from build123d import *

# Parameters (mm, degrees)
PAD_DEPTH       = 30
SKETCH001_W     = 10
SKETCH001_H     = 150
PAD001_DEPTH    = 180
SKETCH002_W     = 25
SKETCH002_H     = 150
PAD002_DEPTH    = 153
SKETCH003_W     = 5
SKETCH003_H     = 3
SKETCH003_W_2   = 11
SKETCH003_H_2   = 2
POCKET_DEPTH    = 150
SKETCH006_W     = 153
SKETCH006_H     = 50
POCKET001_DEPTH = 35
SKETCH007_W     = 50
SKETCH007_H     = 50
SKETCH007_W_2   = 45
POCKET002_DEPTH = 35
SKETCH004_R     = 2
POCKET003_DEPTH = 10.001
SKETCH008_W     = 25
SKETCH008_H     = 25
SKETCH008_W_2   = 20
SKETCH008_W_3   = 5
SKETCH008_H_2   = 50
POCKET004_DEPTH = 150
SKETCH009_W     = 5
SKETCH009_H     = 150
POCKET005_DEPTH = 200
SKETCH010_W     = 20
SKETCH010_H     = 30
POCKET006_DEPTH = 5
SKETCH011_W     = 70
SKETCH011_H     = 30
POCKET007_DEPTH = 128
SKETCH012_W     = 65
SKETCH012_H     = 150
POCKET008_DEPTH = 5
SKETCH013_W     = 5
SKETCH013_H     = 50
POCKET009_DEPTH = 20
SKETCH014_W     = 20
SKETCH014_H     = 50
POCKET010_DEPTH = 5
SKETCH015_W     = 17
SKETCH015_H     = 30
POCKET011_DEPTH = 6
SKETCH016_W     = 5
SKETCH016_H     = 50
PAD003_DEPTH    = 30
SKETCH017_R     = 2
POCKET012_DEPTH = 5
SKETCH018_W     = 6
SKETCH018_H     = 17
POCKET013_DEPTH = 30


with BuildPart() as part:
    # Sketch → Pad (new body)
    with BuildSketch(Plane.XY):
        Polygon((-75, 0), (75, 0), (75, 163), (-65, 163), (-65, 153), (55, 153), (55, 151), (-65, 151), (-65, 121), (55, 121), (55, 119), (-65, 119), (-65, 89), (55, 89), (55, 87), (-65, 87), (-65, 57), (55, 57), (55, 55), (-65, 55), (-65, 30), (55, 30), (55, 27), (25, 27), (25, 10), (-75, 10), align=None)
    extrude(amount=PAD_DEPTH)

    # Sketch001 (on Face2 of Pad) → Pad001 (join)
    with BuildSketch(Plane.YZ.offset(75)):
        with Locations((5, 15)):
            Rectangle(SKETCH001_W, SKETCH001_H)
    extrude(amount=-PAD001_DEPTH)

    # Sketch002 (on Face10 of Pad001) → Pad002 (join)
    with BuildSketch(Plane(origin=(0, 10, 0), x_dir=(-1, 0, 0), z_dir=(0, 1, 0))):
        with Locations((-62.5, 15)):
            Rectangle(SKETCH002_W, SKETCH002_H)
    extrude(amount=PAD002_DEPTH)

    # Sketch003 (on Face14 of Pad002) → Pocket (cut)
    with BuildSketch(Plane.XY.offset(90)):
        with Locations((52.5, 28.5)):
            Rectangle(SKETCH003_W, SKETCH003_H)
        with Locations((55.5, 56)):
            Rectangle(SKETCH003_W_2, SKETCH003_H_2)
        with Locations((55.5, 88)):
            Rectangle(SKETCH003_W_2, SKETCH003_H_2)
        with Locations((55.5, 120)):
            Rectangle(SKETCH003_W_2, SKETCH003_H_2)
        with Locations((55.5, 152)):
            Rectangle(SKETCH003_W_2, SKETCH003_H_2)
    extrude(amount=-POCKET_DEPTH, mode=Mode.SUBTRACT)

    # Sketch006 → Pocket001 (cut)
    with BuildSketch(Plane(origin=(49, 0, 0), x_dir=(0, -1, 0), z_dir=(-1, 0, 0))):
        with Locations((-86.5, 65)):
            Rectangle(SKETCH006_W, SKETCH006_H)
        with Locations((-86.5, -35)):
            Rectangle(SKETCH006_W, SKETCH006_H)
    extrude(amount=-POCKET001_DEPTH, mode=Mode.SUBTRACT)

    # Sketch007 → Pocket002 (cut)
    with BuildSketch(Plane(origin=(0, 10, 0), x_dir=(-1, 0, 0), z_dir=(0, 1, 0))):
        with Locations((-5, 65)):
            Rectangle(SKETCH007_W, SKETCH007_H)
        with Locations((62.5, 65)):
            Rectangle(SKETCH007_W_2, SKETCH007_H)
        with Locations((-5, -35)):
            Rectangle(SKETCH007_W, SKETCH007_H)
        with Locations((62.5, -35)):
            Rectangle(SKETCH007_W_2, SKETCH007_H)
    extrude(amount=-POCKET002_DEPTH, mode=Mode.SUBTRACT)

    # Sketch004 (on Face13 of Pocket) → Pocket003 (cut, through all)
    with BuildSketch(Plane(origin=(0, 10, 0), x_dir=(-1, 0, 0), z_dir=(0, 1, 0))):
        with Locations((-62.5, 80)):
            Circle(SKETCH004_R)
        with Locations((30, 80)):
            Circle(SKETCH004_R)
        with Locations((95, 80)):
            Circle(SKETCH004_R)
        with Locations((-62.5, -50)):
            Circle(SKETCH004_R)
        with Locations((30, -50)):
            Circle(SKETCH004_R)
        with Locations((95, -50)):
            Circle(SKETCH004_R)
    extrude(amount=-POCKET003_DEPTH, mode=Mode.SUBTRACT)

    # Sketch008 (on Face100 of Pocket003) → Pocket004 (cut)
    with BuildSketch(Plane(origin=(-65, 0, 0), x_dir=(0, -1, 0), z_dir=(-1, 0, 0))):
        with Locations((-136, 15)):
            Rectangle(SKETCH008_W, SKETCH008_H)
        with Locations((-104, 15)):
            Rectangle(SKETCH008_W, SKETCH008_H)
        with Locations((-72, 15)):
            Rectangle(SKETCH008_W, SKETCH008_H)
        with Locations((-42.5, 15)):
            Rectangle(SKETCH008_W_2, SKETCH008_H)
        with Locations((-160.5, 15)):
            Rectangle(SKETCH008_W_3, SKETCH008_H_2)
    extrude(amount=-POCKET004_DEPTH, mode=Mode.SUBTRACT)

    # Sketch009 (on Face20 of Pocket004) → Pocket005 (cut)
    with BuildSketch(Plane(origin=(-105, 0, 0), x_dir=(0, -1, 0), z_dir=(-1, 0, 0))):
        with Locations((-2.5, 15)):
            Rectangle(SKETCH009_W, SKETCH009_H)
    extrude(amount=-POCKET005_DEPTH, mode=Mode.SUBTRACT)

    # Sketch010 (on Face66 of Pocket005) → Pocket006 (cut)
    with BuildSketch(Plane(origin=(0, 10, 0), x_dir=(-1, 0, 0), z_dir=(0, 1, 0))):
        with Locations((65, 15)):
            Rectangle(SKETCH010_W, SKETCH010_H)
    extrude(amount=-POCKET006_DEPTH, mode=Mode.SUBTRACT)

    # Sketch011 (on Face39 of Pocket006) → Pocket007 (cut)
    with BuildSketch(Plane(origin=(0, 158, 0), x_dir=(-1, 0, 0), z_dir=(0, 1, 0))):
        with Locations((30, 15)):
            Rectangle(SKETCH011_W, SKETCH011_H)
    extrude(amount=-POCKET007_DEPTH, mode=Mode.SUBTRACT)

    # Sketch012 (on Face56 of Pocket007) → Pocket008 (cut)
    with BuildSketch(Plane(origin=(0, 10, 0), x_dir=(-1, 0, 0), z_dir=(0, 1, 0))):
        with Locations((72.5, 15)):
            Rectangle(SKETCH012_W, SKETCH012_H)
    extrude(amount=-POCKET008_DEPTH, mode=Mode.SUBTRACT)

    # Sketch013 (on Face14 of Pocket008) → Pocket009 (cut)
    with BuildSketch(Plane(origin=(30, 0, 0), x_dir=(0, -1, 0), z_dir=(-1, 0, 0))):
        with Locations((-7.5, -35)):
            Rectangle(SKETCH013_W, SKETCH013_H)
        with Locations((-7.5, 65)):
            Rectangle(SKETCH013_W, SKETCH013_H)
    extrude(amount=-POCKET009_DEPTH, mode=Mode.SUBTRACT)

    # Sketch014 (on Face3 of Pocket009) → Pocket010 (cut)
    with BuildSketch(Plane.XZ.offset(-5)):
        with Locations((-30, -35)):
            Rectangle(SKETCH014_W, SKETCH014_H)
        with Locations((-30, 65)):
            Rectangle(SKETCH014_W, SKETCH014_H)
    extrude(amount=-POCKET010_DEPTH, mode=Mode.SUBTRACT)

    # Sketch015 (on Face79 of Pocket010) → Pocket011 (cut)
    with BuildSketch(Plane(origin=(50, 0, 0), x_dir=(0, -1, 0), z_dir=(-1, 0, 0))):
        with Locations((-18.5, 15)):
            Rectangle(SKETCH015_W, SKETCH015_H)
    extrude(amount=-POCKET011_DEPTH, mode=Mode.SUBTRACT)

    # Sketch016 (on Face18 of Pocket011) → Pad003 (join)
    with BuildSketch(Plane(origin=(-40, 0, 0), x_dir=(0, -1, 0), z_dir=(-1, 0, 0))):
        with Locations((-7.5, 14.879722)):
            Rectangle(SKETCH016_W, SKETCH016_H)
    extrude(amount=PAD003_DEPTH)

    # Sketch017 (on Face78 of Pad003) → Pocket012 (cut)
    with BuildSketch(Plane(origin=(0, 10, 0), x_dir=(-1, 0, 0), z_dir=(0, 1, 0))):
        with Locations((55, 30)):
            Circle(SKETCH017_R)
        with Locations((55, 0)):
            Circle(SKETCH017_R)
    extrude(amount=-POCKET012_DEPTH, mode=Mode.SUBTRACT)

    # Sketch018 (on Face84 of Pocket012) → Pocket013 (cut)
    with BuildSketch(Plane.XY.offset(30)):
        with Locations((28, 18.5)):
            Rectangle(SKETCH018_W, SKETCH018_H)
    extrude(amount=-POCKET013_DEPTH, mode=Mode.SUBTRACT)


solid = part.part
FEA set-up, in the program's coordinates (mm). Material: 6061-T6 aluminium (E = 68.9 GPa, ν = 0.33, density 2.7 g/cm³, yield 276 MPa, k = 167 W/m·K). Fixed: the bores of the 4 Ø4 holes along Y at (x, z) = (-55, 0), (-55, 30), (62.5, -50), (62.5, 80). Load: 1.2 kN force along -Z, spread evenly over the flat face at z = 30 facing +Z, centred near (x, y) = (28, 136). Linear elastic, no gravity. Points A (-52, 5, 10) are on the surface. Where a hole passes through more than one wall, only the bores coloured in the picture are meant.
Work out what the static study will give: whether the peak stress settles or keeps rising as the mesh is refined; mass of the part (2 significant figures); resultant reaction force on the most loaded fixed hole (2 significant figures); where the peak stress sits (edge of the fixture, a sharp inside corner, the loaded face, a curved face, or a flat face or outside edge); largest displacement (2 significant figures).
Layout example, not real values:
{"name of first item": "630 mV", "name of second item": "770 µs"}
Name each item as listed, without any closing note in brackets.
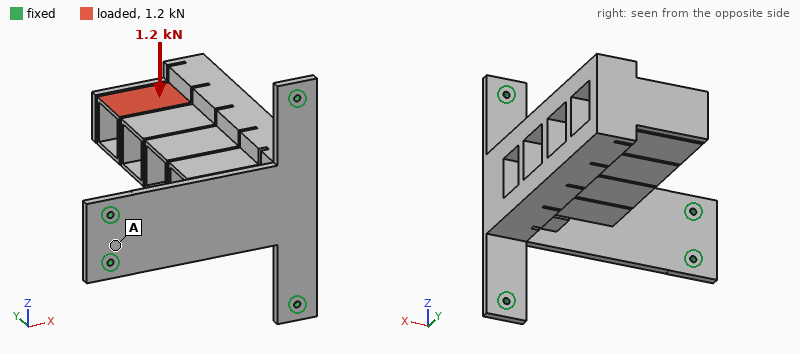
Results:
{"whether the peak stress settles or keeps rising as the mesh is refined": "keeps rising", "mass of the part": "620 g", "resultant reaction force on the most loaded fixed hole": "1.6 kN", "where the peak stress sits": "edge of the fixture", "largest displacement": "2.4 mm"}
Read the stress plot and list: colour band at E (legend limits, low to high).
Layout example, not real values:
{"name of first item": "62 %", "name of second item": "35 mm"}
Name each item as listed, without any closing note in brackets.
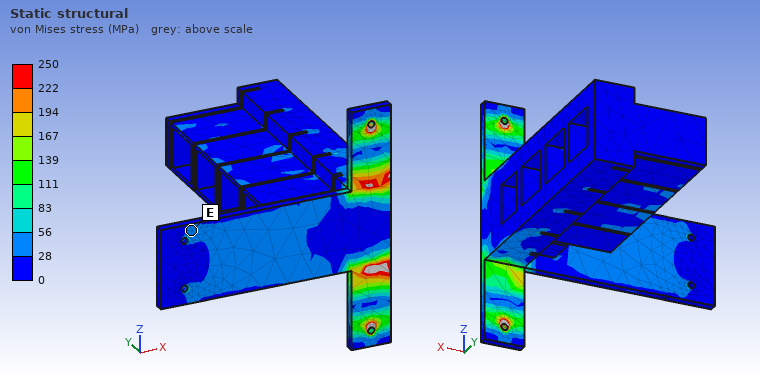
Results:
{"colour band at E": "28 to 56 MPa"}
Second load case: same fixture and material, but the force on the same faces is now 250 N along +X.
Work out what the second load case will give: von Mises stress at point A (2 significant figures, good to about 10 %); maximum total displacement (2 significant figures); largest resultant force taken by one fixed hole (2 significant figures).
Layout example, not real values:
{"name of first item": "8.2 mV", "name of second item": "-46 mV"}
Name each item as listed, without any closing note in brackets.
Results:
{"von Mises stress at point A": "25 MPa", "maximum total displacement": "1.4 mm", "largest resultant force taken by one fixed hole": "220 N"}
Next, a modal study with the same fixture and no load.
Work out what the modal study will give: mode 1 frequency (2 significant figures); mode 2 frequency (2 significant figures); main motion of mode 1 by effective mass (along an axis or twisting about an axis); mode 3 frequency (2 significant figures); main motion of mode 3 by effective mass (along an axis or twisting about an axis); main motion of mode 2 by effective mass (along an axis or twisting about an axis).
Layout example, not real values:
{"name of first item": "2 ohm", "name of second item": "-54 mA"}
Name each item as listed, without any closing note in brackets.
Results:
{"mode 1 frequency": "160 Hz", "mode 2 frequency": "260 Hz", "main motion of mode 1 by effective mass": "along X", "mode 3 frequency": "510 Hz", "main motion of mode 3 by effective mass": "along Y", "main motion of mode 2 by effective mass": "along Z"}
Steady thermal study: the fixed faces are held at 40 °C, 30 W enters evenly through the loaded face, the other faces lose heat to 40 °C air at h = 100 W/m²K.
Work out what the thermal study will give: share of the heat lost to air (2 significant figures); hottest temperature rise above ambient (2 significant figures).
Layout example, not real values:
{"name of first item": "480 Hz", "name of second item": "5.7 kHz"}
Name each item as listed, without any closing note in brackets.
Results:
{"share of the heat lost to air": "98 %", "hottest temperature rise above ambient": "25 K"}
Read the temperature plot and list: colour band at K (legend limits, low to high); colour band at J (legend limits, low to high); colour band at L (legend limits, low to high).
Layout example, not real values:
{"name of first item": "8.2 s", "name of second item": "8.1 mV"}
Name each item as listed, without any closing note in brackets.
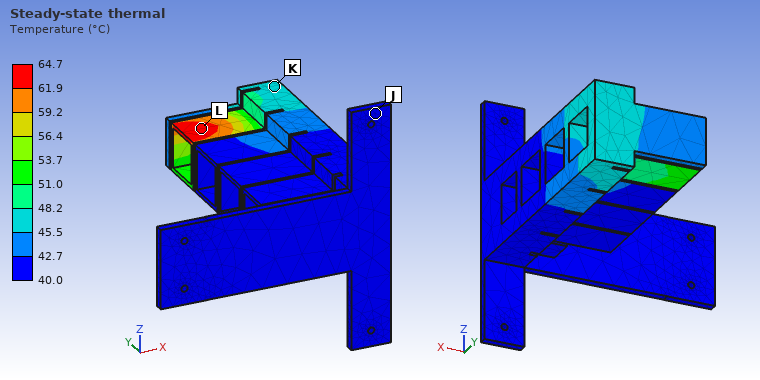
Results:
{"colour band at K": "45.5 to 48.2 °C", "colour band at J": "40.0 to 42.7 °C", "colour band at L": "61.9 to 64.7 °C"}
